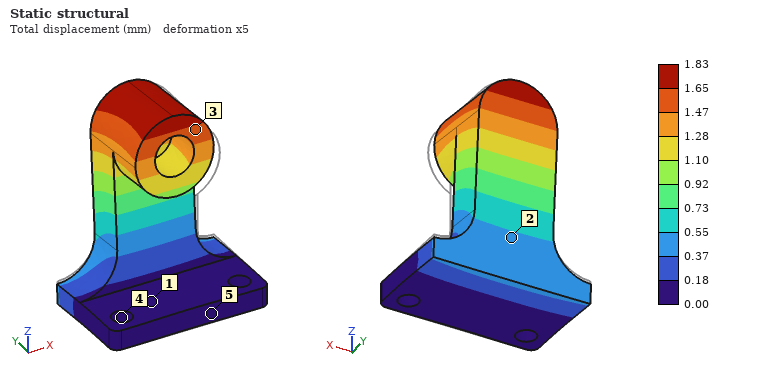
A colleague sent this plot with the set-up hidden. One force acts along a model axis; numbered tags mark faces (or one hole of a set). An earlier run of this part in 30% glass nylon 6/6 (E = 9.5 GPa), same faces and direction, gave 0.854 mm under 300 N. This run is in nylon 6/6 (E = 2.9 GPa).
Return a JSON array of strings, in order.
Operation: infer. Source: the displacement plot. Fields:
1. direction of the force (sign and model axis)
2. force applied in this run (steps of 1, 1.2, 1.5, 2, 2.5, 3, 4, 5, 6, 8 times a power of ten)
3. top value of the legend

["+Y", "200 N", "1.83 mm"]
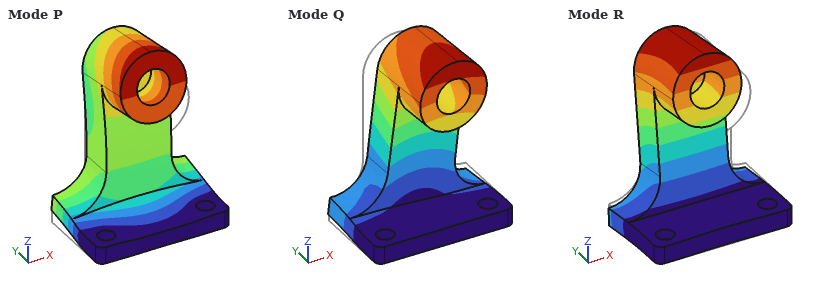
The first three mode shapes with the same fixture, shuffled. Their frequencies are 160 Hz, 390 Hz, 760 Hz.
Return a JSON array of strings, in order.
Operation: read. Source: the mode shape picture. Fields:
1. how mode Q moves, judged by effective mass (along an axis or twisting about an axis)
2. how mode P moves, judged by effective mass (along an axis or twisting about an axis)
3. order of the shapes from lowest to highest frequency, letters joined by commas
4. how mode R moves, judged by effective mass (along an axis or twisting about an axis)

["along X", "along Z", "R, Q, P", "along Y"]
